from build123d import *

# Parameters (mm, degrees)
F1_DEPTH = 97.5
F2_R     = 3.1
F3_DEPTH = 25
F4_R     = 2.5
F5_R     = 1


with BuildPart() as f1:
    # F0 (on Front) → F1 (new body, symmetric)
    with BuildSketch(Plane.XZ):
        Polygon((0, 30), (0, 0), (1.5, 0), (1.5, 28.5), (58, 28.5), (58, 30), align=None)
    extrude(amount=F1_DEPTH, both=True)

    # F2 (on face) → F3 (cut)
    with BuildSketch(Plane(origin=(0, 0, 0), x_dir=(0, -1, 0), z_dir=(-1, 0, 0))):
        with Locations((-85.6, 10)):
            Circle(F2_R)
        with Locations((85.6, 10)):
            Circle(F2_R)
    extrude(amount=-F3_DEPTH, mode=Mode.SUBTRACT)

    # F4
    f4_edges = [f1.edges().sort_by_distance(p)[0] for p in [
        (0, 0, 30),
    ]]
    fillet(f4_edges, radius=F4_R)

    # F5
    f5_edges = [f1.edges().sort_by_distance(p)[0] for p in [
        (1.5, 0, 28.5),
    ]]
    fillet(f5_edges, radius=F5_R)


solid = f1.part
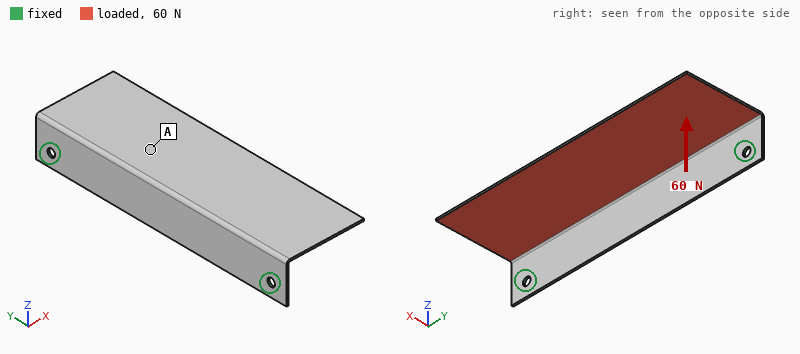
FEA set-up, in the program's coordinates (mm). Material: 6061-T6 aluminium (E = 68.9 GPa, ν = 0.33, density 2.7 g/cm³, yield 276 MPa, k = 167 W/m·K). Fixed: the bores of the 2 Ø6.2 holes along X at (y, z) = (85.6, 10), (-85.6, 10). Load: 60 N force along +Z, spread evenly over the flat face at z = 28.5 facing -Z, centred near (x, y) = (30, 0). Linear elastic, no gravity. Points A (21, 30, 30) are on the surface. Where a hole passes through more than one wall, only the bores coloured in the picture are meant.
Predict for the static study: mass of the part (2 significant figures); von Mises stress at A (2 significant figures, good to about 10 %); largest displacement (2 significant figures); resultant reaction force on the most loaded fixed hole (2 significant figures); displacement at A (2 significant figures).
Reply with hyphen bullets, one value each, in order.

- 67 g
- 7.8 MPa
- 1.7 mm
- 38 N
- 0.55 mm
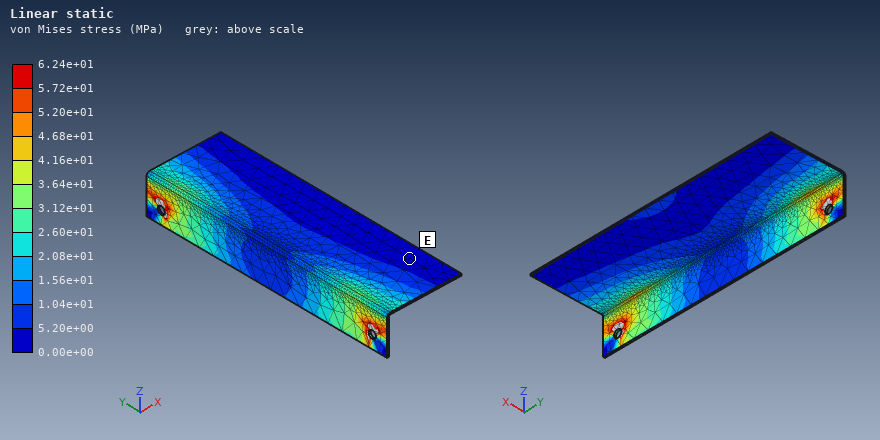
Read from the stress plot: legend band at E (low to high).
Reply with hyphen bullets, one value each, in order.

- 0.00e+00 to 5.20e+00 MPa
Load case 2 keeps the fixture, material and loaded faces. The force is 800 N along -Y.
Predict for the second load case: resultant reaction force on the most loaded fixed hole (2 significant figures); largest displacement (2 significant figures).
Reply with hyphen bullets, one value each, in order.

- 430 N
- 1.2 mm
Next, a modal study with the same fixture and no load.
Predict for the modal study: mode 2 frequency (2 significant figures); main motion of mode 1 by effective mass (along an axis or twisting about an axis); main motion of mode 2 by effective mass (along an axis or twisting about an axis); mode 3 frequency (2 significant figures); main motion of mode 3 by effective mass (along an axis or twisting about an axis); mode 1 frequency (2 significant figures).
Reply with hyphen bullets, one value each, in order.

- 330 Hz
- along Z
- twisting about X
- 510 Hz
- along X
- 180 Hz
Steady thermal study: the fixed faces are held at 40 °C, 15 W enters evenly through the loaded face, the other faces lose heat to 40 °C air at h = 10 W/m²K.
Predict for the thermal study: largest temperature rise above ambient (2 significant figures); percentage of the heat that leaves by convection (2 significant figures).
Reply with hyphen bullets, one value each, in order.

- 26 K
- 27 %
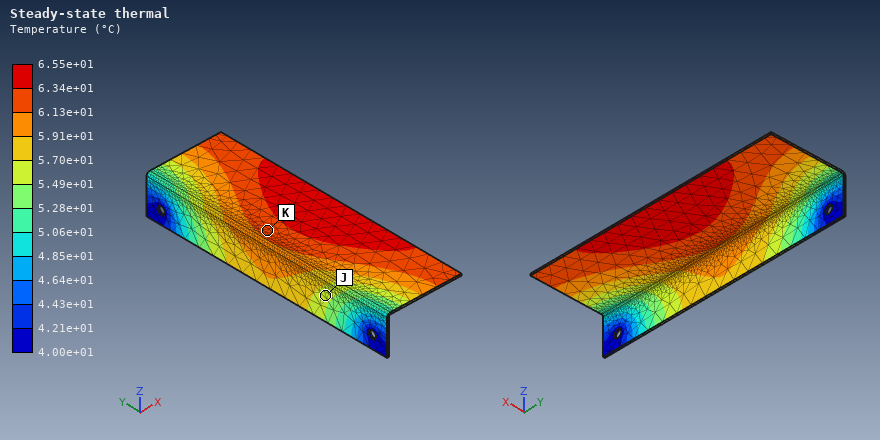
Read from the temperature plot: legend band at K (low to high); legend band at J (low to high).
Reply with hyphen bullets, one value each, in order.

- 6.13e+01 to 6.34e+01 °C
- 5.49e+01 to 5.70e+01 °C
